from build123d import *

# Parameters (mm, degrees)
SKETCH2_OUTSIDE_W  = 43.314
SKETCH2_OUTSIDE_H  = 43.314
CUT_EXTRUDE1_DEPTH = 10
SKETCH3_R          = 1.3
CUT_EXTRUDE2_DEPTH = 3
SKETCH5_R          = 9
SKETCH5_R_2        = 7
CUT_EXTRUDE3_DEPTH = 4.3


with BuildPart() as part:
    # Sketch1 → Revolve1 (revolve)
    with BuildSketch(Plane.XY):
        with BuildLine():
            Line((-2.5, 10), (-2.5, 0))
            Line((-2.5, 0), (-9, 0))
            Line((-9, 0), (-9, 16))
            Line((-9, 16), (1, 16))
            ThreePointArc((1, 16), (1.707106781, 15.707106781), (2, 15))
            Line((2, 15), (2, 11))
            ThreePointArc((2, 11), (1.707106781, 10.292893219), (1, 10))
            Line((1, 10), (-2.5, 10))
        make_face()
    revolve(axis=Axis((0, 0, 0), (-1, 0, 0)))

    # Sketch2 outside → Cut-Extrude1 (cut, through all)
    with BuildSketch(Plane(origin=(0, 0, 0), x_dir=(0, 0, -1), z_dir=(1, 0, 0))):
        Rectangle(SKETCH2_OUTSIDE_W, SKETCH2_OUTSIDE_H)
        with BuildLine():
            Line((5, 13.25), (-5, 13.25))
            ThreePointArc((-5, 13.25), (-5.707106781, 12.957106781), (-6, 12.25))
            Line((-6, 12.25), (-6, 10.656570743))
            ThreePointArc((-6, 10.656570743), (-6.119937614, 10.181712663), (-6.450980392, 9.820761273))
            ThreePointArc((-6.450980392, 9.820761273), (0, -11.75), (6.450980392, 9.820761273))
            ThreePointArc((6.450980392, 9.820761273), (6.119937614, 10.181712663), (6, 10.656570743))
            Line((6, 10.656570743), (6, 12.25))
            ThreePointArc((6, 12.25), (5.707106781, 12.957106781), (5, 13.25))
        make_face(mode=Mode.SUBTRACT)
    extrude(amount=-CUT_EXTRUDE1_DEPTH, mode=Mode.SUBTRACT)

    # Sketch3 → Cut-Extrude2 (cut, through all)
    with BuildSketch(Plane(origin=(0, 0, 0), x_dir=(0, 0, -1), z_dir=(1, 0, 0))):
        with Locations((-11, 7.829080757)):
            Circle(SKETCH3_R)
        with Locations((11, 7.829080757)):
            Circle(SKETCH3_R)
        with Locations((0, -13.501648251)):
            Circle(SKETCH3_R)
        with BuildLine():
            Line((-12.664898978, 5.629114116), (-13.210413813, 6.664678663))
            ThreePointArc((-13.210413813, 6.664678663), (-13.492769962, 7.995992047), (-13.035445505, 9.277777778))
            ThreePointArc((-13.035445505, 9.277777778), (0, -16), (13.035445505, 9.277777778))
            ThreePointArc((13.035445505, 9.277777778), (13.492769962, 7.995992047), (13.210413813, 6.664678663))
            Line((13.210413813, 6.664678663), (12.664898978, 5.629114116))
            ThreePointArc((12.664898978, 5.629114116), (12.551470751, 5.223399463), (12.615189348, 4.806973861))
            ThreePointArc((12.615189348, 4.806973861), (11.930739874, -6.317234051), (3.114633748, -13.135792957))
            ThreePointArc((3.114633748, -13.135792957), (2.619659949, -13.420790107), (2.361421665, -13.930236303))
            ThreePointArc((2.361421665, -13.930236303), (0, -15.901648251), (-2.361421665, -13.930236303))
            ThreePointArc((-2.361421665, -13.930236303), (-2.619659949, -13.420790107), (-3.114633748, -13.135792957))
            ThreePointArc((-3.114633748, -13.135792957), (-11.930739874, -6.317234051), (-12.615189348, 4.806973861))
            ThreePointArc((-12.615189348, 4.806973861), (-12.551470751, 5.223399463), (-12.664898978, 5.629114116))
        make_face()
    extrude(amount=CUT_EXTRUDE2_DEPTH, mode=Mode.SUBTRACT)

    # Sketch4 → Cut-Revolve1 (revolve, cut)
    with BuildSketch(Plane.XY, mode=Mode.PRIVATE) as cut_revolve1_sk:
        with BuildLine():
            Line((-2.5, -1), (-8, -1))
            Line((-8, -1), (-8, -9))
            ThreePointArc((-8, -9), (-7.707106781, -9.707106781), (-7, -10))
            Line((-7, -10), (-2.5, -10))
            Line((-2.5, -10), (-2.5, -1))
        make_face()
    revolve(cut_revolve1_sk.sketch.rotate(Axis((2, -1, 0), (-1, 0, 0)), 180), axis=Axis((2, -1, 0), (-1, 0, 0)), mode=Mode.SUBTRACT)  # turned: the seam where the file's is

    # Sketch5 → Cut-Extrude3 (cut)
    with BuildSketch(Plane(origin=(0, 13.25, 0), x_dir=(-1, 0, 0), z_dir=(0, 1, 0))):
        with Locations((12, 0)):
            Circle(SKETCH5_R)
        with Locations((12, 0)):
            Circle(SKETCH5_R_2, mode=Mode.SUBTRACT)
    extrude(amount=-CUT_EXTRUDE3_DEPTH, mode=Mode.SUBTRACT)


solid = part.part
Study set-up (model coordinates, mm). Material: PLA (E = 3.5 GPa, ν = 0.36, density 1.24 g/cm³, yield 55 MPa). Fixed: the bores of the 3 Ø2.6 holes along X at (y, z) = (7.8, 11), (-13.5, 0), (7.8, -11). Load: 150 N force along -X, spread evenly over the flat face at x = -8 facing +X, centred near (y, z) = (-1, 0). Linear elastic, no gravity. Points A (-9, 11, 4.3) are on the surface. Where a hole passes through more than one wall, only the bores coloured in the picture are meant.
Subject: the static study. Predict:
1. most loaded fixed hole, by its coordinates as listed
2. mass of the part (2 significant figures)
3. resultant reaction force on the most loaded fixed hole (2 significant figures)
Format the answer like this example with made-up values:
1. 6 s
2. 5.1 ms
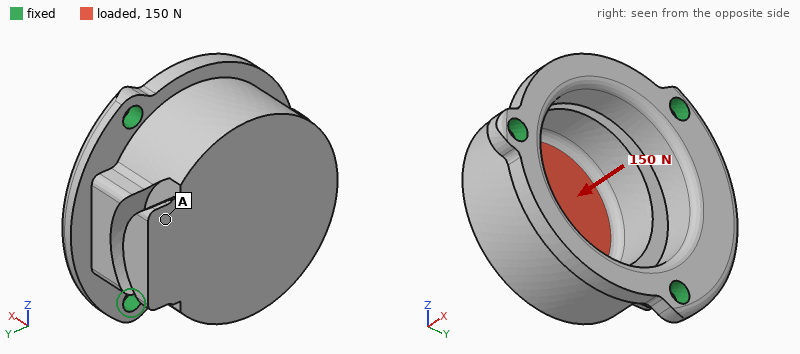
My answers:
1. (-13.5, 0)
2. 3.1 g
3. 66 N
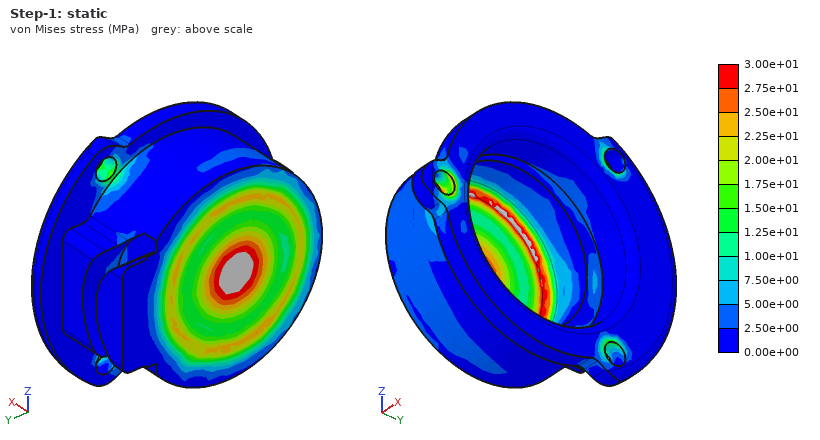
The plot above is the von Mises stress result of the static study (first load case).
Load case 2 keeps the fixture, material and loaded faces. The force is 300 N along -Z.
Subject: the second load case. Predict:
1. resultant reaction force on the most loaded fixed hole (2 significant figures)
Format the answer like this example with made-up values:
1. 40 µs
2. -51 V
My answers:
1. 170 N
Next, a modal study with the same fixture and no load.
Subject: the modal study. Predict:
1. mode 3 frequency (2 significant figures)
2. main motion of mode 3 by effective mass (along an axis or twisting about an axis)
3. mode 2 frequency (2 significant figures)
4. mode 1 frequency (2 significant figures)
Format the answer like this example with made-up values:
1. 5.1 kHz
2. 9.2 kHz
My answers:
1. 8600 Hz
2. along X
3. 7100 Hz
4. 7000 Hz
